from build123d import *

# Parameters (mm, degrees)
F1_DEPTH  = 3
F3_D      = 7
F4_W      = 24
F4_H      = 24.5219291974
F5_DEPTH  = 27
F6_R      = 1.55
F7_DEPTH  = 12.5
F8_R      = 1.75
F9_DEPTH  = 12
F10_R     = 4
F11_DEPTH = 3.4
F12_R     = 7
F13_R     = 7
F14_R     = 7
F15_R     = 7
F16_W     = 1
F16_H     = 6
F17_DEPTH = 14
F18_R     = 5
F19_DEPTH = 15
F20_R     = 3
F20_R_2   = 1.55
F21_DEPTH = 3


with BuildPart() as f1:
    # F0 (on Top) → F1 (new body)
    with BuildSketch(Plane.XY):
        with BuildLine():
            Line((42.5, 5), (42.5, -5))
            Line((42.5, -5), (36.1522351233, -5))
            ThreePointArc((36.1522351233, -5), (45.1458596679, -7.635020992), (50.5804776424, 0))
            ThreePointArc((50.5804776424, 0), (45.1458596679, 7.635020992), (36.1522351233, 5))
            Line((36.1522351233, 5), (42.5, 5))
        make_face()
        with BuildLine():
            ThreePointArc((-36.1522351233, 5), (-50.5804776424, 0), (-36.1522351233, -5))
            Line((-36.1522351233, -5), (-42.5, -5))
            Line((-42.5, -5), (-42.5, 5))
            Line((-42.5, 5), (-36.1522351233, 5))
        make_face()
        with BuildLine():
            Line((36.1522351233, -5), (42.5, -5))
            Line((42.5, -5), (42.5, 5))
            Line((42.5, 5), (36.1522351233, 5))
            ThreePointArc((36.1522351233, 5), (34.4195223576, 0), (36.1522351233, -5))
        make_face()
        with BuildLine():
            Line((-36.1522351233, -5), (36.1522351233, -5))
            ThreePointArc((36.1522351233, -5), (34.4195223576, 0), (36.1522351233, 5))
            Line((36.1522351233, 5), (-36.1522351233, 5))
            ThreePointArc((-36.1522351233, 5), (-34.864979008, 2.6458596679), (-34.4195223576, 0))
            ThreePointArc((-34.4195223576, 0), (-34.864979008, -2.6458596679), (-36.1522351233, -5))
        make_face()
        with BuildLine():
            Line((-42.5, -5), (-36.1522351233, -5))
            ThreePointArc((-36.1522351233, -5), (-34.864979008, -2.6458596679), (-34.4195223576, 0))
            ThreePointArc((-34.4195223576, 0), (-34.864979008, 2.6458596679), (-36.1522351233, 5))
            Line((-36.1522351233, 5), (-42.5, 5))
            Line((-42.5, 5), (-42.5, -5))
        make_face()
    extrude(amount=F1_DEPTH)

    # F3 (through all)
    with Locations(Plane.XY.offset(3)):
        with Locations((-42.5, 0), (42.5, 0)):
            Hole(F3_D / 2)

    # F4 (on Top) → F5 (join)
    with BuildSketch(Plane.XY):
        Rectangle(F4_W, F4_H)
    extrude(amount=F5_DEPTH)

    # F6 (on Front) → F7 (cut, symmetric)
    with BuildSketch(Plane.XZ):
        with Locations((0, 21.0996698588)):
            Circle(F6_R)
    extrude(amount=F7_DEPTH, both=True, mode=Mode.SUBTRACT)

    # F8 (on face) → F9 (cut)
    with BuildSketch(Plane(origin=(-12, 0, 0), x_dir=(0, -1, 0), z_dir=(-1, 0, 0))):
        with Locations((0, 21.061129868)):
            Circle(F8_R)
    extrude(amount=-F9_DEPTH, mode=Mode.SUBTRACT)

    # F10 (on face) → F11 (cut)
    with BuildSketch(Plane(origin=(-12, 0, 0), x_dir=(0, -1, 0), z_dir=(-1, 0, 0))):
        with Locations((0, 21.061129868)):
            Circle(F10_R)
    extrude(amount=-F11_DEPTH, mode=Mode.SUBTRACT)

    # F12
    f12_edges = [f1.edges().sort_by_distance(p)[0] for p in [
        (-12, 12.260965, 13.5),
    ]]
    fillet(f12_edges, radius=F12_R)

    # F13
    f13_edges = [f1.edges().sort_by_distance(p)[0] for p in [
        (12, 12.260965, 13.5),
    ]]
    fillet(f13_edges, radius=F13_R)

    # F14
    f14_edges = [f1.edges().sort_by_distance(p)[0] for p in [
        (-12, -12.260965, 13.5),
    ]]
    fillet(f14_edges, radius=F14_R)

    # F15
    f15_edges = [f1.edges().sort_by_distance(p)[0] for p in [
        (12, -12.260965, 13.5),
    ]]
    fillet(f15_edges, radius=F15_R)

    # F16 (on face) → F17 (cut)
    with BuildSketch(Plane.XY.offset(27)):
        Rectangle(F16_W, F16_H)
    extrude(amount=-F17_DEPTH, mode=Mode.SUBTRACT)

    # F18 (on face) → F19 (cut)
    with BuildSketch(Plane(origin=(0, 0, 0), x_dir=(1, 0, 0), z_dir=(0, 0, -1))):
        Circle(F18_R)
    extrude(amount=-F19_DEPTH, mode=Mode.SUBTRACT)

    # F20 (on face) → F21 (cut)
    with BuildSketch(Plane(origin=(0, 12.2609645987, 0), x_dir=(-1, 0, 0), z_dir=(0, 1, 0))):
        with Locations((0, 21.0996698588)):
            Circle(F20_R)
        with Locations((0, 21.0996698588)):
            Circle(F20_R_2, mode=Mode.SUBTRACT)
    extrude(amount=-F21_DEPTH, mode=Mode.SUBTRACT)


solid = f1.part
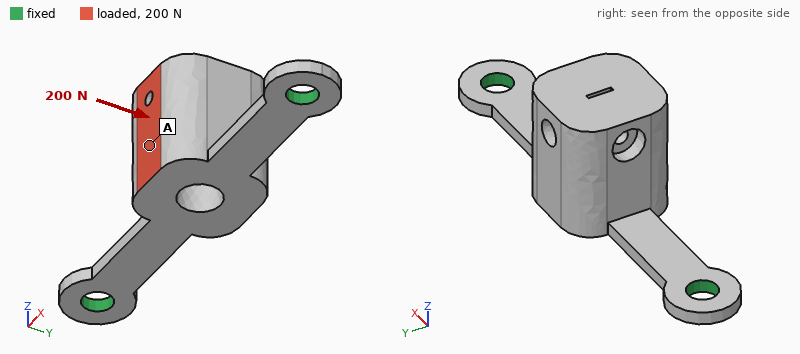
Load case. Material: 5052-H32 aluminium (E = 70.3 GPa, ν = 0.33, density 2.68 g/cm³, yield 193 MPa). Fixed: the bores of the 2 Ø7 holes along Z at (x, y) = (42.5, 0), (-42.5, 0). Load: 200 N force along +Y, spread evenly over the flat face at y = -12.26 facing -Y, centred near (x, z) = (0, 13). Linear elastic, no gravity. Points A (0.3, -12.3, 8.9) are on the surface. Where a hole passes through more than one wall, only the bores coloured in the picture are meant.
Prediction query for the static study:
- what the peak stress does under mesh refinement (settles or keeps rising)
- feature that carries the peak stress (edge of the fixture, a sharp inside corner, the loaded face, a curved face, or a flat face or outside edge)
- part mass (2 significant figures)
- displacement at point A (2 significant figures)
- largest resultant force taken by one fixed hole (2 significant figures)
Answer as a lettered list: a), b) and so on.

a) keeps rising
b) a sharp inside corner
c) 41 g
d) 0.23 mm
e) 100 N
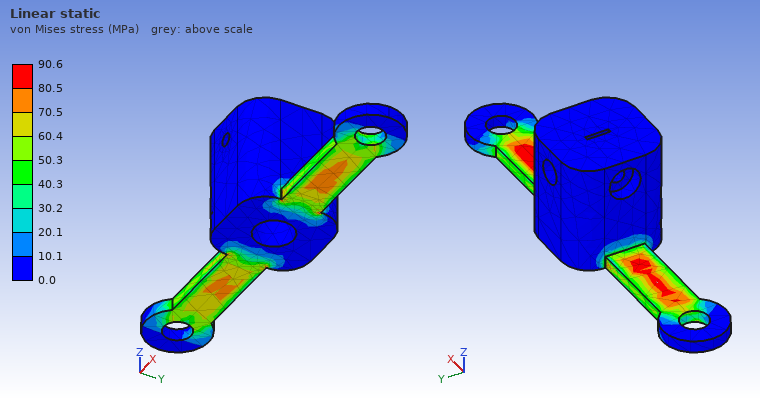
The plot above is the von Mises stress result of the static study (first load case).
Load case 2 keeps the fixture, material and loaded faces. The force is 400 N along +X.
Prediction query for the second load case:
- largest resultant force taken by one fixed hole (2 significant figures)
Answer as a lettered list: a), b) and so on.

a) 230 N
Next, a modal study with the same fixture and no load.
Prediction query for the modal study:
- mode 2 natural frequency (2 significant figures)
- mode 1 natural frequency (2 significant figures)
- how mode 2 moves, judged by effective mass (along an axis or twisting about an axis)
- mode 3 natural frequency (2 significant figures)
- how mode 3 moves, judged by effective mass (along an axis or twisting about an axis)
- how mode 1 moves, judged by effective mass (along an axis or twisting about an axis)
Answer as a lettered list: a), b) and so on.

a) 1100 Hz
b) 640 Hz
c) along Z
d) 1700 Hz
e) along X
f) along Y
